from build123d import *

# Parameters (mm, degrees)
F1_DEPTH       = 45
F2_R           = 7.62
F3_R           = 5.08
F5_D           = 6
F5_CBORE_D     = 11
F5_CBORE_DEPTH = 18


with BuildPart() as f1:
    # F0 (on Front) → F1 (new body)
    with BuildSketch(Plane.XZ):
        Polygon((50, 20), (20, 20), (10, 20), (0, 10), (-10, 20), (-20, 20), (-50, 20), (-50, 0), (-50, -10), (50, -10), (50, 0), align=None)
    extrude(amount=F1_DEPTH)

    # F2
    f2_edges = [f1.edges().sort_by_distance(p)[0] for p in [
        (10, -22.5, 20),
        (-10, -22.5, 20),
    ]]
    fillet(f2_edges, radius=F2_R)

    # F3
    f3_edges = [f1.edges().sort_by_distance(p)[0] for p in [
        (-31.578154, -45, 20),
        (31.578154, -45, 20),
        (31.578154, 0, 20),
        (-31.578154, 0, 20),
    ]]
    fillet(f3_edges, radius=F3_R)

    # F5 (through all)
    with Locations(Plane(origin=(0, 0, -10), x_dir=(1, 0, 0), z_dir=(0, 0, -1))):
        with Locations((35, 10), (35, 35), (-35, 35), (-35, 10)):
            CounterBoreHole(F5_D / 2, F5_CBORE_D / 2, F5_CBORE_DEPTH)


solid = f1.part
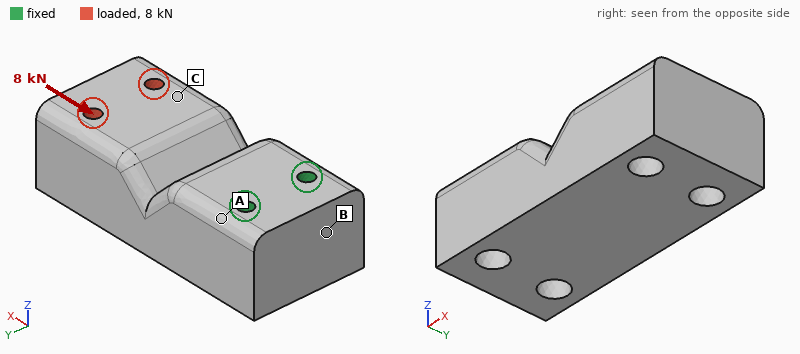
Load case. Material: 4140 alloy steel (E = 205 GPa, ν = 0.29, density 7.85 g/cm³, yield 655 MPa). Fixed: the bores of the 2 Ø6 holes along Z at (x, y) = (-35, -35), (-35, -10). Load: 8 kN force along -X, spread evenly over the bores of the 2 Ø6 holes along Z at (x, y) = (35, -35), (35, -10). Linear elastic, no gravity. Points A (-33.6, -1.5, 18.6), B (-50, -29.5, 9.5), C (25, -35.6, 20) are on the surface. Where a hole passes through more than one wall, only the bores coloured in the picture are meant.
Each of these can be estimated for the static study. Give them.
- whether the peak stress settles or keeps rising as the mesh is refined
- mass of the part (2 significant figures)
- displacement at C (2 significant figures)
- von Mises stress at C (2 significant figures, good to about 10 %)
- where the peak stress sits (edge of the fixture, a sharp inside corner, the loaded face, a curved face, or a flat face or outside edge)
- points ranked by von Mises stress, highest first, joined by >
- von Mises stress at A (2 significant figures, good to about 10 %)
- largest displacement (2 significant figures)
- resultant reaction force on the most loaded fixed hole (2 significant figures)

keeps rising
950 g
15 µm
18 MPa
a sharp inside corner
C > A > B
9.6 MPa
25 µm
4.0 kN
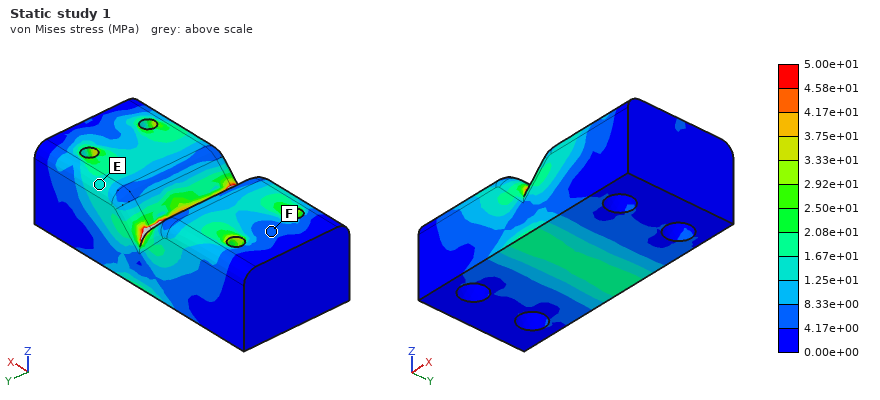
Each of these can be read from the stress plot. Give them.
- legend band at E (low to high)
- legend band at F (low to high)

1.25e+01 to 1.67e+01 MPa
4.17e+00 to 8.33e+00 MPa
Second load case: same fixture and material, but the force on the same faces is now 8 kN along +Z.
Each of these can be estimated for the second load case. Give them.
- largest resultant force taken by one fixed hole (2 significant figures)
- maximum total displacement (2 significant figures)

4.3 kN
0.25 mm
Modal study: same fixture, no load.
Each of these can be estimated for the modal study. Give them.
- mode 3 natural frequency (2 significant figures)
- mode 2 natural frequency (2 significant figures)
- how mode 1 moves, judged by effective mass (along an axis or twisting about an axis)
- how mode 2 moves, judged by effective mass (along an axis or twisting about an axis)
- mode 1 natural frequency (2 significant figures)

6800 Hz
3200 Hz
along Z
along Y
1600 Hz
